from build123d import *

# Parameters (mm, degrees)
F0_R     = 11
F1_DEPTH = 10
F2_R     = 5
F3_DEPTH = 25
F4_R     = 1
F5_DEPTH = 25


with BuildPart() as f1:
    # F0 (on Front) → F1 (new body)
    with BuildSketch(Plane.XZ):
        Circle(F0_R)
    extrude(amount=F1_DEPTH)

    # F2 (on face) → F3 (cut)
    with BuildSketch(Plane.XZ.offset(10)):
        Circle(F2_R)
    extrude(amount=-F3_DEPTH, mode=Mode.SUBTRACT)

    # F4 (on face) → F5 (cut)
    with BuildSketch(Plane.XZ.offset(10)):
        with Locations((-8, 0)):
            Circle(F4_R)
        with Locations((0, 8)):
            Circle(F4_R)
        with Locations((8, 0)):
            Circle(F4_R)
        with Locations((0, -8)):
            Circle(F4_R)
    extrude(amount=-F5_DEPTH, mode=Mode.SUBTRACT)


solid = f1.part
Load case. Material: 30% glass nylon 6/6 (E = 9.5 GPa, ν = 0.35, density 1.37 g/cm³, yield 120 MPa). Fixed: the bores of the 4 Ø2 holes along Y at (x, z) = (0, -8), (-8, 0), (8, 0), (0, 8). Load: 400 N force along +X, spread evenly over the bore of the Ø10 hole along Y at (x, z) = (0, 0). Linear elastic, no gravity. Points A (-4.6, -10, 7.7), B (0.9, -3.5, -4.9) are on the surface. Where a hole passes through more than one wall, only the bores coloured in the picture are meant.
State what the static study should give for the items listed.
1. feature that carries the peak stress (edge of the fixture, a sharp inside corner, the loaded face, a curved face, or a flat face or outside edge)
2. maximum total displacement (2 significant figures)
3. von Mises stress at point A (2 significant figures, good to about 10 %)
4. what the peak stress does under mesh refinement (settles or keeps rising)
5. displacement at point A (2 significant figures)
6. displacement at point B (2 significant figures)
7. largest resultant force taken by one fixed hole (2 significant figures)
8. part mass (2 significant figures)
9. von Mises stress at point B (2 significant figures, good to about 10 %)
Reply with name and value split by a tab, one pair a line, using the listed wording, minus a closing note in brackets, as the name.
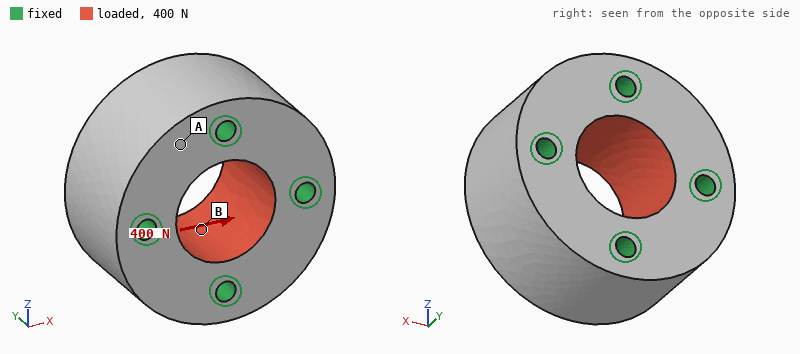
feature that carries the peak stress	edge of the fixture
maximum total displacement	1.2 µm
von Mises stress at point A	0.85 MPa
what the peak stress does under mesh refinement	keeps rising
displacement at point A	0.61 µm
displacement at point B	1.1 µm
largest resultant force taken by one fixed hole	100 N
part mass	4.0 g
von Mises stress at point B	2.2 MPa
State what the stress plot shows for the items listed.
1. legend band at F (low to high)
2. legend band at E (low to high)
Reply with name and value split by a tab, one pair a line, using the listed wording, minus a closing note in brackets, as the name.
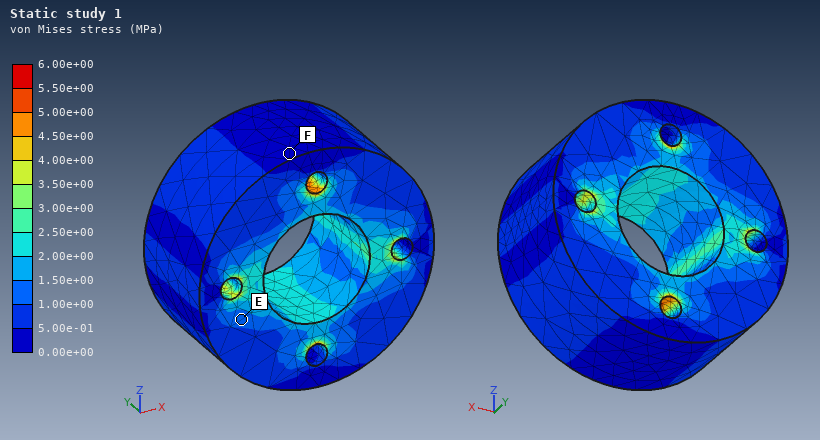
legend band at F	0.00e+00 to 5.00e-01 MPa
legend band at E	1.00e+00 to 1.50e+00 MPa
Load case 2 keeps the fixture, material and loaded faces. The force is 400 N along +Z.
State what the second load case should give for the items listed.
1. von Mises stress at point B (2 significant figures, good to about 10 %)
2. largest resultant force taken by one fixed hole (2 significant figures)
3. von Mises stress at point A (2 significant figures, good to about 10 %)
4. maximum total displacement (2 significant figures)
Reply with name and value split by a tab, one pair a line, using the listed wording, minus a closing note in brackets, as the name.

von Mises stress at point B	2.0 MPa
largest resultant force taken by one fixed hole	100 N
von Mises stress at point A	0.78 MPa
maximum total displacement	1.2 µm
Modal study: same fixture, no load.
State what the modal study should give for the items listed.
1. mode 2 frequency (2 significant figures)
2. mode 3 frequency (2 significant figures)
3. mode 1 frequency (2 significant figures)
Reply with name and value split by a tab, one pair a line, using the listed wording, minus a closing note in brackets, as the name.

mode 2 frequency	53 kHz
mode 3 frequency	53 kHz
mode 1 frequency	51 kHz
